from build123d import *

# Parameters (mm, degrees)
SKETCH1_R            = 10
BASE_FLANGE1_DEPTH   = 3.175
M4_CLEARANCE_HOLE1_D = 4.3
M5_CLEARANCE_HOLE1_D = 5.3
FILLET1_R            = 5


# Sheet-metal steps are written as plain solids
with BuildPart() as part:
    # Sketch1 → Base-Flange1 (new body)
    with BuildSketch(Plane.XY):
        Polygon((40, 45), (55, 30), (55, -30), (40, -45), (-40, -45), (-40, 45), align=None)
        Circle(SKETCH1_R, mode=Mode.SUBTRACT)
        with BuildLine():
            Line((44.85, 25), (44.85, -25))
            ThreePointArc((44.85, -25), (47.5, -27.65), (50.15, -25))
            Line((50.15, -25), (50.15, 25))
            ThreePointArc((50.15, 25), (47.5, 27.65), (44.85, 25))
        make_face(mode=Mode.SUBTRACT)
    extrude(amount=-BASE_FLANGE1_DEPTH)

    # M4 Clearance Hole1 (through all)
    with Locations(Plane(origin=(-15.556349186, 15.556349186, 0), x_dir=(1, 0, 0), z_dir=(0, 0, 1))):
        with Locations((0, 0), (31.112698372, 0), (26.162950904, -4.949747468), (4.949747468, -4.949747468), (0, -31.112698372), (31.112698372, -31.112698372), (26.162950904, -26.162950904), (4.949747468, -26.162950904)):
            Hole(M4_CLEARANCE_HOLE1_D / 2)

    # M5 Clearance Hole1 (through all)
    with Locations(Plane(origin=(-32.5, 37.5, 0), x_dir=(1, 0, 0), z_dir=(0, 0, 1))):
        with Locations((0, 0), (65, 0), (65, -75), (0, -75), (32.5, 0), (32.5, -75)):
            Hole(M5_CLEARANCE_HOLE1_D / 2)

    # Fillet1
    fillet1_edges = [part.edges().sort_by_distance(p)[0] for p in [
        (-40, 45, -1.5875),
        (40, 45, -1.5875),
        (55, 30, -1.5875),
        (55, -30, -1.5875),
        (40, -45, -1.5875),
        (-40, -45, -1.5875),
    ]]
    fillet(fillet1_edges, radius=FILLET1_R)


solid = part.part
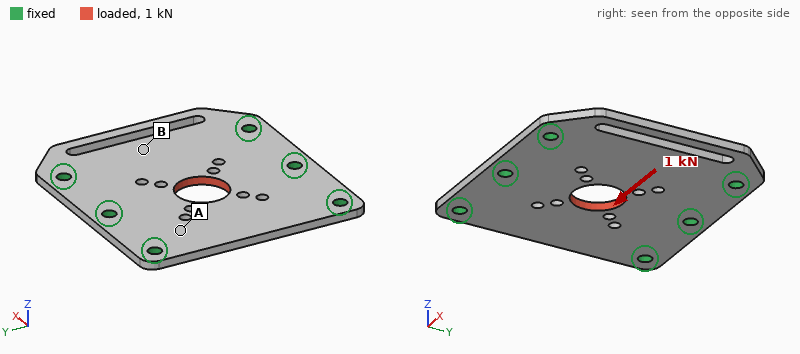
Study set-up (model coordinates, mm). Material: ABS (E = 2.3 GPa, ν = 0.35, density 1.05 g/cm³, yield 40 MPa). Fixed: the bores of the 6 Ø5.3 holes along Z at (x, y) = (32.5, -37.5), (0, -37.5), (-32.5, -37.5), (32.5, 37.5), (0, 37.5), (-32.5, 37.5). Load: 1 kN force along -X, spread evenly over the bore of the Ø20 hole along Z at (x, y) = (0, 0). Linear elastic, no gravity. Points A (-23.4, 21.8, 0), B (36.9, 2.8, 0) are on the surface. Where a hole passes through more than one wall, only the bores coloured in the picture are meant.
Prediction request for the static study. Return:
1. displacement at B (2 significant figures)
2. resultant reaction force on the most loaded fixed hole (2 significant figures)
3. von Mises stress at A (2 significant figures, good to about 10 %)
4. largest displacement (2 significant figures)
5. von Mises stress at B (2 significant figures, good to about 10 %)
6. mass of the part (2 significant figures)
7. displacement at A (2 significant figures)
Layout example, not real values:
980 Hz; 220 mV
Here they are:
0.070 mm; 200 N; 3.7 MPa; 0.11 mm; 1.8 MPa; 25 g; 0.043 mm
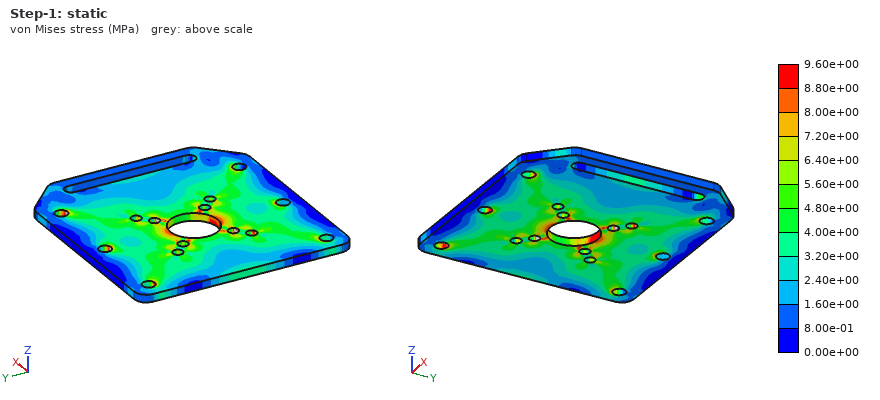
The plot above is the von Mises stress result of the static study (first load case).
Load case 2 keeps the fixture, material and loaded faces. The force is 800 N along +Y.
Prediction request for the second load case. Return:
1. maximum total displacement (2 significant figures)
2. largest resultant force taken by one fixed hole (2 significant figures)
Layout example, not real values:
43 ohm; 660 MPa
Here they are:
58 µm; 200 N
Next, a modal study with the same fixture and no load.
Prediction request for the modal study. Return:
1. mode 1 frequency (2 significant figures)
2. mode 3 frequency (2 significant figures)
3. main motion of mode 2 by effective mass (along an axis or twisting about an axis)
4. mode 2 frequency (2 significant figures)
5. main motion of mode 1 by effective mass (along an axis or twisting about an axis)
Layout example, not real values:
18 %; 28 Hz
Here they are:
790 Hz; 1100 Hz; along Z; 910 Hz; along Z
